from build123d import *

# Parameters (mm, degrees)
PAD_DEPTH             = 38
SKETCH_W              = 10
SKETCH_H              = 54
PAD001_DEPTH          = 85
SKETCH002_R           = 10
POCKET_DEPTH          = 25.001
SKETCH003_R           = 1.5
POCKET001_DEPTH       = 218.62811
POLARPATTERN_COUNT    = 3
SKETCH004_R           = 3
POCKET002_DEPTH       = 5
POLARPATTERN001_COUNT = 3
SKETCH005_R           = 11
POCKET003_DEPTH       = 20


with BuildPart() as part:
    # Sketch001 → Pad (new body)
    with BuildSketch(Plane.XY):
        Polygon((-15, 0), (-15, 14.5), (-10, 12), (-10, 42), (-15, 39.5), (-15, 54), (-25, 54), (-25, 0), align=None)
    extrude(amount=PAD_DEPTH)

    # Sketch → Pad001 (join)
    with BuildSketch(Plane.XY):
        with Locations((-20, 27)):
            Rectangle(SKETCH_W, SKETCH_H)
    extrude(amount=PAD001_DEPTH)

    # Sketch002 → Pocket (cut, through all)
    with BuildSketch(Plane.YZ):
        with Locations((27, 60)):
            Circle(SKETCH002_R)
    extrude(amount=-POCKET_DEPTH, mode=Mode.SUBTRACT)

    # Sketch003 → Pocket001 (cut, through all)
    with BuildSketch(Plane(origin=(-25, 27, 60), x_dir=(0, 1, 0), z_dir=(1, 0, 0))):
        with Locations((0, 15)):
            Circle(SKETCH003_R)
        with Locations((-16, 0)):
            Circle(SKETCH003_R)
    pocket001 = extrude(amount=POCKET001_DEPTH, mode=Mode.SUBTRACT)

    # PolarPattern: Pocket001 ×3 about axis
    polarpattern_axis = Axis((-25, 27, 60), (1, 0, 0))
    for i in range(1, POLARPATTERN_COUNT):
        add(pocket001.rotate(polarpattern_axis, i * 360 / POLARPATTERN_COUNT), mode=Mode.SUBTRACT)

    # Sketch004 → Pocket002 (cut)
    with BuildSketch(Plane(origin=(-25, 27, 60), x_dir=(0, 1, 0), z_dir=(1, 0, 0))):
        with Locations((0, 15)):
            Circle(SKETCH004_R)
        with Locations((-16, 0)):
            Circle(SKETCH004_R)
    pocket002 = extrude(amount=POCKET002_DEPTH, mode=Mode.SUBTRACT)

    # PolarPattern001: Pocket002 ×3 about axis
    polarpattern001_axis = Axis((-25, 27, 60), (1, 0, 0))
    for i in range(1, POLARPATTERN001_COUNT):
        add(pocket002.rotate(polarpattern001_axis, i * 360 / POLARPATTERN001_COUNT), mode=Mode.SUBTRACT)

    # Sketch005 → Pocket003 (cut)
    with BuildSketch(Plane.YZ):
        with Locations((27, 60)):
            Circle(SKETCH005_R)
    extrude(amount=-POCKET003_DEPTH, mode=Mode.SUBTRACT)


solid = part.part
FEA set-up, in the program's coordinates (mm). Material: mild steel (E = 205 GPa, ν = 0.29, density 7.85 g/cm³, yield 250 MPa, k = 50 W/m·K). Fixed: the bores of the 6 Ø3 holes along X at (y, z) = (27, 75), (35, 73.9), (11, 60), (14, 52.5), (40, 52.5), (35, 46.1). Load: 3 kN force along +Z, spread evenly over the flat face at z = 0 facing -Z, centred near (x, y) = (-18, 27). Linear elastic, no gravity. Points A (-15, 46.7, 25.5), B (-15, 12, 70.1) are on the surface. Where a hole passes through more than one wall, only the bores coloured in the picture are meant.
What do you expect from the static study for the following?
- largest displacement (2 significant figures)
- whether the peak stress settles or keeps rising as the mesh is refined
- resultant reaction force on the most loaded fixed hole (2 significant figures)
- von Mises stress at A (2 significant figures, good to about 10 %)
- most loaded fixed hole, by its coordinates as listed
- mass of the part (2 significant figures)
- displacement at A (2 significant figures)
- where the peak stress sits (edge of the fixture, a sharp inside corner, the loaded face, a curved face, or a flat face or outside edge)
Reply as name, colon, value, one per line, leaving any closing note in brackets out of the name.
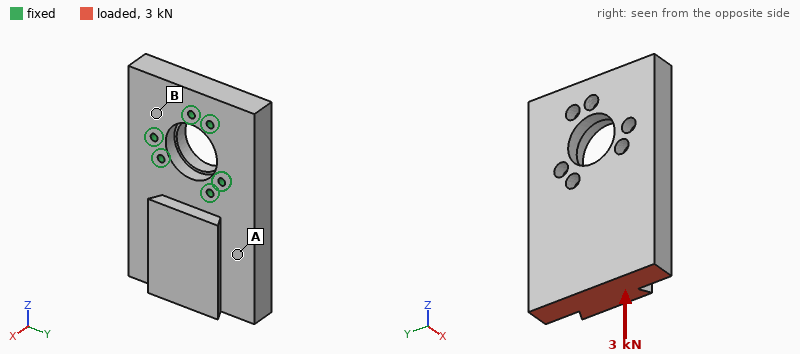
largest displacement: 2.8 µm
whether the peak stress settles or keeps rising as the mesh is refined: keeps rising
resultant reaction force on the most loaded fixed hole: 1.0 kN
von Mises stress at A: 5.6 MPa
most loaded fixed hole, by its coordinates as listed: (35, 46.1)
mass of the part: 370 g
displacement at A: 1.3 µm
where the peak stress sits: edge of the fixture
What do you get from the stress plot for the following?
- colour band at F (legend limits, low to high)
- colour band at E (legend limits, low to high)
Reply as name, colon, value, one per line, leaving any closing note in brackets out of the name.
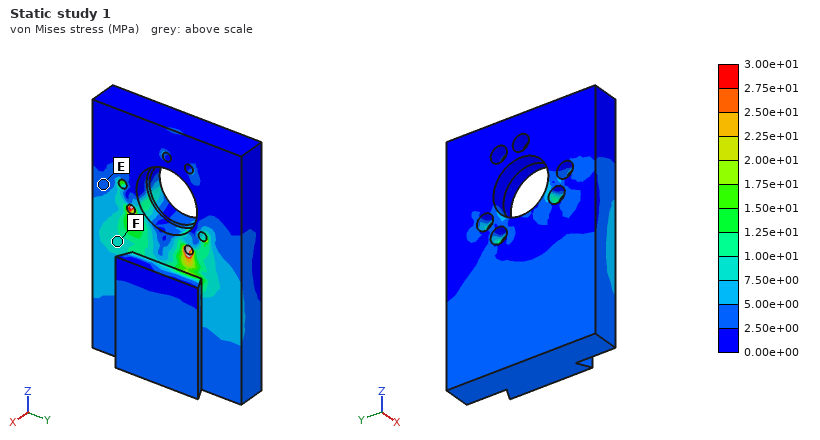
colour band at F: 7.50e+00 to 1.00e+01 MPa
colour band at E: 2.50e+00 to 5.00e+00 MPa
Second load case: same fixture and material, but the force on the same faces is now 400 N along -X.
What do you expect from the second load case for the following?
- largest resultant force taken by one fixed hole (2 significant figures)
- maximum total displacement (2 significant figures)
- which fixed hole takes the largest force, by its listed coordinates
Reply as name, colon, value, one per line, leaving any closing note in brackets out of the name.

largest resultant force taken by one fixed hole: 1.0 kN
maximum total displacement: 28 µm
which fixed hole takes the largest force, by its listed coordinates: (35, 46.1)
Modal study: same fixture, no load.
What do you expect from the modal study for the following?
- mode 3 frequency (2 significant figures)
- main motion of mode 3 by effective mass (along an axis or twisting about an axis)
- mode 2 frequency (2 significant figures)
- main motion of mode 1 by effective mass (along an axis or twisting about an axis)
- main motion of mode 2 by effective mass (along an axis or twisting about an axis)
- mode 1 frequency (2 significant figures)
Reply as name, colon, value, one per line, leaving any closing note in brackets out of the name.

mode 3 frequency: 7500 Hz
main motion of mode 3 by effective mass: along Y
mode 2 frequency: 6000 Hz
main motion of mode 1 by effective mass: along X
main motion of mode 2 by effective mass: twisting about Z
mode 1 frequency: 2200 Hz
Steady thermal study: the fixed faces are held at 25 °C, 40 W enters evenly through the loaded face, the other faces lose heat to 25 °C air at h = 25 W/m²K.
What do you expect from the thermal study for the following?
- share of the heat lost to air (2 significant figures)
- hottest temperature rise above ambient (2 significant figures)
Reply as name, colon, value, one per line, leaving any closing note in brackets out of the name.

share of the heat lost to air: 18 %
hottest temperature rise above ambient: 65 K
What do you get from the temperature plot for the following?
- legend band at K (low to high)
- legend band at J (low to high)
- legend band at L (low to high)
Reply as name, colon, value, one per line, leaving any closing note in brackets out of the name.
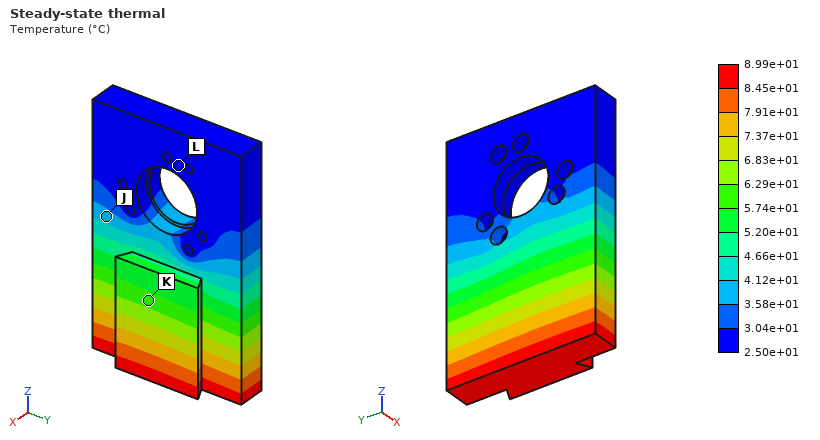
legend band at K: 5.74e+01 to 6.29e+01 °C
legend band at J: 3.58e+01 to 4.12e+01 °C
legend band at L: 2.50e+01 to 3.04e+01 °C
